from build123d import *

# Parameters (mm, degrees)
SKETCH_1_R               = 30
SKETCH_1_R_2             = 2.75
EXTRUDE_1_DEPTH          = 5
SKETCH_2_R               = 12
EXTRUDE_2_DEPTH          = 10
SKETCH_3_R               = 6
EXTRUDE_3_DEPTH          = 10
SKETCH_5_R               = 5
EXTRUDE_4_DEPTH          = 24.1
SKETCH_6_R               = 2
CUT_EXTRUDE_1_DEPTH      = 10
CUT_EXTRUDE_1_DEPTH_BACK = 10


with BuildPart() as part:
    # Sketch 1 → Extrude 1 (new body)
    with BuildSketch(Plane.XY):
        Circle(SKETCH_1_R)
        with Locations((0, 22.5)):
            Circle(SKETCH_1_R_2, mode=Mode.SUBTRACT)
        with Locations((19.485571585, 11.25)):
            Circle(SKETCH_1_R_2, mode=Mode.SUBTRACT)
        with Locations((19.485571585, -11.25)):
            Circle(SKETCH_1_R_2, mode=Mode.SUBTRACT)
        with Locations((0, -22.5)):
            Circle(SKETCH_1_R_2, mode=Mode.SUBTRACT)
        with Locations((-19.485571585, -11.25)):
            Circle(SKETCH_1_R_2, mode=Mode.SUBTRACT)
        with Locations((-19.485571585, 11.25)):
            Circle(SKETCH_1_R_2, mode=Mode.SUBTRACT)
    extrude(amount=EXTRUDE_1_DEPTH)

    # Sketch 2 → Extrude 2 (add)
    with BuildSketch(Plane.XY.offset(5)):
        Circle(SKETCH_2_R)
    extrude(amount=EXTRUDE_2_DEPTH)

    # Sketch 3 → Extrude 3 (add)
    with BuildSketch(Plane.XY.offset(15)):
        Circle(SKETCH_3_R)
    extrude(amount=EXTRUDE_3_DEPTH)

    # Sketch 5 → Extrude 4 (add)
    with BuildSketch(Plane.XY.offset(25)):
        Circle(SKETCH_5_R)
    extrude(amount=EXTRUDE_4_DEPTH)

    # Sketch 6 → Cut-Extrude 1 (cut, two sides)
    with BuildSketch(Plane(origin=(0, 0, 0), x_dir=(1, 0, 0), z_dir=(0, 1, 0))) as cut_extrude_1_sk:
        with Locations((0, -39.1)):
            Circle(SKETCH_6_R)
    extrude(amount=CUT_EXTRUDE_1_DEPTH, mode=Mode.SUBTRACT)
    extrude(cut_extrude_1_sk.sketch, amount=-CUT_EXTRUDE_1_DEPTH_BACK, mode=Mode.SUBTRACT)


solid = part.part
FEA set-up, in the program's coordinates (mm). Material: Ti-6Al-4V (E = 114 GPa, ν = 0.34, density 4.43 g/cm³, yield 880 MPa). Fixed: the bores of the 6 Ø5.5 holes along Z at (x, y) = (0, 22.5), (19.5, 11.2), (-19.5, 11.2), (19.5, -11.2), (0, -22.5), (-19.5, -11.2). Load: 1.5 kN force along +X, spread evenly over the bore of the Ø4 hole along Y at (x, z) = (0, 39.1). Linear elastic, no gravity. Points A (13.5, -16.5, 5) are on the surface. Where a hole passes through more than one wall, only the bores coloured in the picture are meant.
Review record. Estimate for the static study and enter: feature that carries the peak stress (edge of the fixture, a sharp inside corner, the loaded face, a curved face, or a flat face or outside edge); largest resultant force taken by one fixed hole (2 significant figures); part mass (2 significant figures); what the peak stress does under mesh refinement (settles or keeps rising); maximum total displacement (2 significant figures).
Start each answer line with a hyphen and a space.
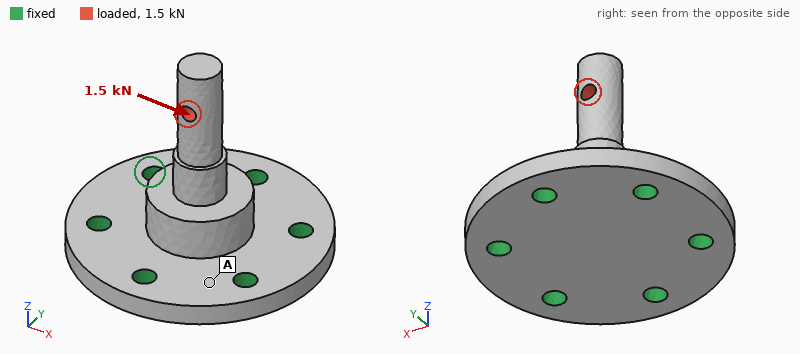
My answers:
- a sharp inside corner
- 980 N
- 92 g
- keeps rising
- 0.20 mm
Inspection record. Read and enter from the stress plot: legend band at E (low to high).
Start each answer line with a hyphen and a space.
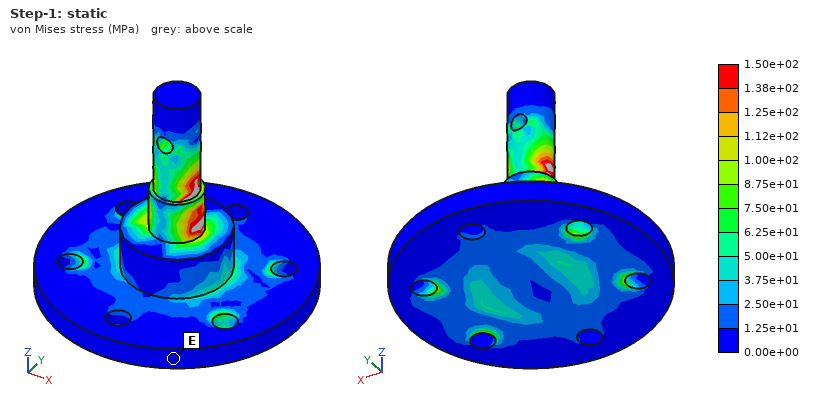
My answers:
- 0.00e+00 to 1.25e+01 MPa
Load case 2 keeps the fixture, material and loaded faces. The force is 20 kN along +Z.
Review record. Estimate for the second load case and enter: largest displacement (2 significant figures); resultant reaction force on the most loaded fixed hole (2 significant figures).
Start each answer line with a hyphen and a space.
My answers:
- 0.10 mm
- 3.7 kN
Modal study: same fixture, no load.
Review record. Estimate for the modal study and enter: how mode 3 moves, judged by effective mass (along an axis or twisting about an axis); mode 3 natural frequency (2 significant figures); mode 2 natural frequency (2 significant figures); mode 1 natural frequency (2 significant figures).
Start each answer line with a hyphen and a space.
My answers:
- along Z
- 16 kHz
- 6100 Hz
- 6100 Hz
